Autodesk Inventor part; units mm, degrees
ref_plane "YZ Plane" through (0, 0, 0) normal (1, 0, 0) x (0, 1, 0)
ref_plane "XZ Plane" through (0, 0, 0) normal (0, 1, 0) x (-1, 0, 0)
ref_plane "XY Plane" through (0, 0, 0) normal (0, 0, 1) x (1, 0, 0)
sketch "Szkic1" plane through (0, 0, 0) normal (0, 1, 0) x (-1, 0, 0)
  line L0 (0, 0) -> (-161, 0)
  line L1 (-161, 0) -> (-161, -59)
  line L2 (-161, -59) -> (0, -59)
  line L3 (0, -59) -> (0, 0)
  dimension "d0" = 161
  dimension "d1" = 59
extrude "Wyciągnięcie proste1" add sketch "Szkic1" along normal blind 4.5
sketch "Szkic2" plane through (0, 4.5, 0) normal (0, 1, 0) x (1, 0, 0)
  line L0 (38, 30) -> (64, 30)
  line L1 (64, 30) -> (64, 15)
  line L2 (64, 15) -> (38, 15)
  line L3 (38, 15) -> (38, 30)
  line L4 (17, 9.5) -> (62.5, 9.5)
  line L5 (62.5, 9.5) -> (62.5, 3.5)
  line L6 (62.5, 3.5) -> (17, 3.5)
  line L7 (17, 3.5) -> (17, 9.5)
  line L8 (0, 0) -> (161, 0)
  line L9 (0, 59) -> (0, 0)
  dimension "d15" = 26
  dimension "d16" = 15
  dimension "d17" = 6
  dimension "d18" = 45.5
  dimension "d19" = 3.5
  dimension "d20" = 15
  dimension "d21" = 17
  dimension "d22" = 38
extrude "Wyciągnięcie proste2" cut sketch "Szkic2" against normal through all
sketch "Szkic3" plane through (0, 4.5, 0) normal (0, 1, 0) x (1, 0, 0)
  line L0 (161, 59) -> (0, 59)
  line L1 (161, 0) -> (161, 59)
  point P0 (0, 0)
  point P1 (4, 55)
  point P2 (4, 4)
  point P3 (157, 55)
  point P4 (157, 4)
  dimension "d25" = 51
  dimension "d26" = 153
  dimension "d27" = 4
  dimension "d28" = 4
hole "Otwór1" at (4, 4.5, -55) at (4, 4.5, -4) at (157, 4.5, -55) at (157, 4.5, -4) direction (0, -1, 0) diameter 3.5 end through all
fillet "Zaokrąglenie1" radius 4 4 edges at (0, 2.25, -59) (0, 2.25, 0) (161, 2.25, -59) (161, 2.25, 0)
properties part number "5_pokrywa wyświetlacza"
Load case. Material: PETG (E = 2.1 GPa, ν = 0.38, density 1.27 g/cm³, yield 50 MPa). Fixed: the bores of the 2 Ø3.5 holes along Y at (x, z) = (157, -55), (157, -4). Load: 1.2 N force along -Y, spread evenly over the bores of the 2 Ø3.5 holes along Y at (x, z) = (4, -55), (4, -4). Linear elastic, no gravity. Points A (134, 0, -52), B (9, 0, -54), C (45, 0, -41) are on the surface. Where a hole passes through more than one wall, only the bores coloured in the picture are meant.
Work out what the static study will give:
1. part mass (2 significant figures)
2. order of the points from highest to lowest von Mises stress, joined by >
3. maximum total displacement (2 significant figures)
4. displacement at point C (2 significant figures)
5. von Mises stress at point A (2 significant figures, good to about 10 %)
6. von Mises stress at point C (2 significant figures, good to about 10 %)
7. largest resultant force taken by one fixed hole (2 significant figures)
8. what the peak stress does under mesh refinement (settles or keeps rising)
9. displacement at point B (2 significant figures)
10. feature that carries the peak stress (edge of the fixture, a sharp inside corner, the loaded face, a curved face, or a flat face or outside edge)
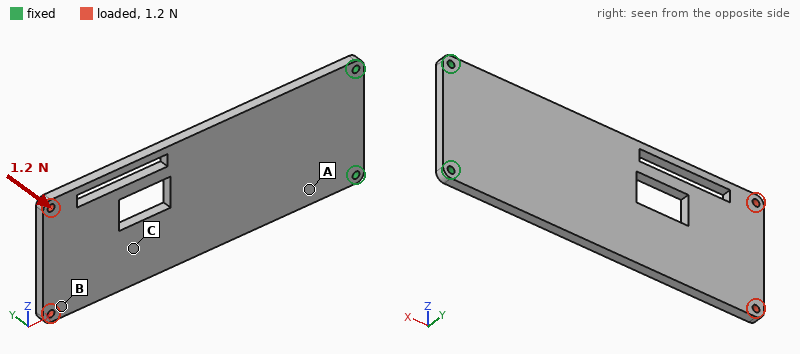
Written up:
50 g
A > C > B
1.9 mm
1.1 mm
0.81 MPa
0.37 MPa
0.60 N
keeps rising
1.7 mm
edge of the fixture
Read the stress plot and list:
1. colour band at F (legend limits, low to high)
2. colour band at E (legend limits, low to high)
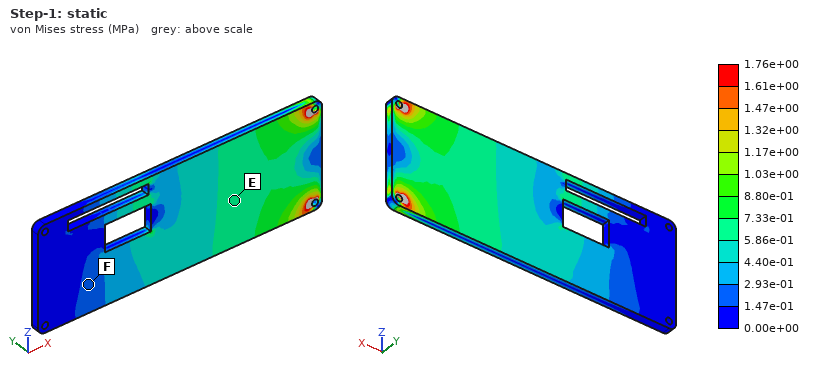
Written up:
1.47e-01 to 2.93e-01 MPa
5.86e-01 to 7.33e-01 MPa
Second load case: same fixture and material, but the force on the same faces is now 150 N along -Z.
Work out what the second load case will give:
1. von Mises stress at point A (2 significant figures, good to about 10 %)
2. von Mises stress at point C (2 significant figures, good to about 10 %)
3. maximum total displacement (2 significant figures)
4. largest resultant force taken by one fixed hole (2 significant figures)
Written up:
5.8 MPa
2.9 MPa
1.6 mm
460 N
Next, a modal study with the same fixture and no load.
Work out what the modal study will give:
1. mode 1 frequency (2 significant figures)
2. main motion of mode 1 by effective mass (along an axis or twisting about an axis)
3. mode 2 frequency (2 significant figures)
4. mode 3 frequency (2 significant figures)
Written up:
36 Hz
along Y
210 Hz
210 Hz
